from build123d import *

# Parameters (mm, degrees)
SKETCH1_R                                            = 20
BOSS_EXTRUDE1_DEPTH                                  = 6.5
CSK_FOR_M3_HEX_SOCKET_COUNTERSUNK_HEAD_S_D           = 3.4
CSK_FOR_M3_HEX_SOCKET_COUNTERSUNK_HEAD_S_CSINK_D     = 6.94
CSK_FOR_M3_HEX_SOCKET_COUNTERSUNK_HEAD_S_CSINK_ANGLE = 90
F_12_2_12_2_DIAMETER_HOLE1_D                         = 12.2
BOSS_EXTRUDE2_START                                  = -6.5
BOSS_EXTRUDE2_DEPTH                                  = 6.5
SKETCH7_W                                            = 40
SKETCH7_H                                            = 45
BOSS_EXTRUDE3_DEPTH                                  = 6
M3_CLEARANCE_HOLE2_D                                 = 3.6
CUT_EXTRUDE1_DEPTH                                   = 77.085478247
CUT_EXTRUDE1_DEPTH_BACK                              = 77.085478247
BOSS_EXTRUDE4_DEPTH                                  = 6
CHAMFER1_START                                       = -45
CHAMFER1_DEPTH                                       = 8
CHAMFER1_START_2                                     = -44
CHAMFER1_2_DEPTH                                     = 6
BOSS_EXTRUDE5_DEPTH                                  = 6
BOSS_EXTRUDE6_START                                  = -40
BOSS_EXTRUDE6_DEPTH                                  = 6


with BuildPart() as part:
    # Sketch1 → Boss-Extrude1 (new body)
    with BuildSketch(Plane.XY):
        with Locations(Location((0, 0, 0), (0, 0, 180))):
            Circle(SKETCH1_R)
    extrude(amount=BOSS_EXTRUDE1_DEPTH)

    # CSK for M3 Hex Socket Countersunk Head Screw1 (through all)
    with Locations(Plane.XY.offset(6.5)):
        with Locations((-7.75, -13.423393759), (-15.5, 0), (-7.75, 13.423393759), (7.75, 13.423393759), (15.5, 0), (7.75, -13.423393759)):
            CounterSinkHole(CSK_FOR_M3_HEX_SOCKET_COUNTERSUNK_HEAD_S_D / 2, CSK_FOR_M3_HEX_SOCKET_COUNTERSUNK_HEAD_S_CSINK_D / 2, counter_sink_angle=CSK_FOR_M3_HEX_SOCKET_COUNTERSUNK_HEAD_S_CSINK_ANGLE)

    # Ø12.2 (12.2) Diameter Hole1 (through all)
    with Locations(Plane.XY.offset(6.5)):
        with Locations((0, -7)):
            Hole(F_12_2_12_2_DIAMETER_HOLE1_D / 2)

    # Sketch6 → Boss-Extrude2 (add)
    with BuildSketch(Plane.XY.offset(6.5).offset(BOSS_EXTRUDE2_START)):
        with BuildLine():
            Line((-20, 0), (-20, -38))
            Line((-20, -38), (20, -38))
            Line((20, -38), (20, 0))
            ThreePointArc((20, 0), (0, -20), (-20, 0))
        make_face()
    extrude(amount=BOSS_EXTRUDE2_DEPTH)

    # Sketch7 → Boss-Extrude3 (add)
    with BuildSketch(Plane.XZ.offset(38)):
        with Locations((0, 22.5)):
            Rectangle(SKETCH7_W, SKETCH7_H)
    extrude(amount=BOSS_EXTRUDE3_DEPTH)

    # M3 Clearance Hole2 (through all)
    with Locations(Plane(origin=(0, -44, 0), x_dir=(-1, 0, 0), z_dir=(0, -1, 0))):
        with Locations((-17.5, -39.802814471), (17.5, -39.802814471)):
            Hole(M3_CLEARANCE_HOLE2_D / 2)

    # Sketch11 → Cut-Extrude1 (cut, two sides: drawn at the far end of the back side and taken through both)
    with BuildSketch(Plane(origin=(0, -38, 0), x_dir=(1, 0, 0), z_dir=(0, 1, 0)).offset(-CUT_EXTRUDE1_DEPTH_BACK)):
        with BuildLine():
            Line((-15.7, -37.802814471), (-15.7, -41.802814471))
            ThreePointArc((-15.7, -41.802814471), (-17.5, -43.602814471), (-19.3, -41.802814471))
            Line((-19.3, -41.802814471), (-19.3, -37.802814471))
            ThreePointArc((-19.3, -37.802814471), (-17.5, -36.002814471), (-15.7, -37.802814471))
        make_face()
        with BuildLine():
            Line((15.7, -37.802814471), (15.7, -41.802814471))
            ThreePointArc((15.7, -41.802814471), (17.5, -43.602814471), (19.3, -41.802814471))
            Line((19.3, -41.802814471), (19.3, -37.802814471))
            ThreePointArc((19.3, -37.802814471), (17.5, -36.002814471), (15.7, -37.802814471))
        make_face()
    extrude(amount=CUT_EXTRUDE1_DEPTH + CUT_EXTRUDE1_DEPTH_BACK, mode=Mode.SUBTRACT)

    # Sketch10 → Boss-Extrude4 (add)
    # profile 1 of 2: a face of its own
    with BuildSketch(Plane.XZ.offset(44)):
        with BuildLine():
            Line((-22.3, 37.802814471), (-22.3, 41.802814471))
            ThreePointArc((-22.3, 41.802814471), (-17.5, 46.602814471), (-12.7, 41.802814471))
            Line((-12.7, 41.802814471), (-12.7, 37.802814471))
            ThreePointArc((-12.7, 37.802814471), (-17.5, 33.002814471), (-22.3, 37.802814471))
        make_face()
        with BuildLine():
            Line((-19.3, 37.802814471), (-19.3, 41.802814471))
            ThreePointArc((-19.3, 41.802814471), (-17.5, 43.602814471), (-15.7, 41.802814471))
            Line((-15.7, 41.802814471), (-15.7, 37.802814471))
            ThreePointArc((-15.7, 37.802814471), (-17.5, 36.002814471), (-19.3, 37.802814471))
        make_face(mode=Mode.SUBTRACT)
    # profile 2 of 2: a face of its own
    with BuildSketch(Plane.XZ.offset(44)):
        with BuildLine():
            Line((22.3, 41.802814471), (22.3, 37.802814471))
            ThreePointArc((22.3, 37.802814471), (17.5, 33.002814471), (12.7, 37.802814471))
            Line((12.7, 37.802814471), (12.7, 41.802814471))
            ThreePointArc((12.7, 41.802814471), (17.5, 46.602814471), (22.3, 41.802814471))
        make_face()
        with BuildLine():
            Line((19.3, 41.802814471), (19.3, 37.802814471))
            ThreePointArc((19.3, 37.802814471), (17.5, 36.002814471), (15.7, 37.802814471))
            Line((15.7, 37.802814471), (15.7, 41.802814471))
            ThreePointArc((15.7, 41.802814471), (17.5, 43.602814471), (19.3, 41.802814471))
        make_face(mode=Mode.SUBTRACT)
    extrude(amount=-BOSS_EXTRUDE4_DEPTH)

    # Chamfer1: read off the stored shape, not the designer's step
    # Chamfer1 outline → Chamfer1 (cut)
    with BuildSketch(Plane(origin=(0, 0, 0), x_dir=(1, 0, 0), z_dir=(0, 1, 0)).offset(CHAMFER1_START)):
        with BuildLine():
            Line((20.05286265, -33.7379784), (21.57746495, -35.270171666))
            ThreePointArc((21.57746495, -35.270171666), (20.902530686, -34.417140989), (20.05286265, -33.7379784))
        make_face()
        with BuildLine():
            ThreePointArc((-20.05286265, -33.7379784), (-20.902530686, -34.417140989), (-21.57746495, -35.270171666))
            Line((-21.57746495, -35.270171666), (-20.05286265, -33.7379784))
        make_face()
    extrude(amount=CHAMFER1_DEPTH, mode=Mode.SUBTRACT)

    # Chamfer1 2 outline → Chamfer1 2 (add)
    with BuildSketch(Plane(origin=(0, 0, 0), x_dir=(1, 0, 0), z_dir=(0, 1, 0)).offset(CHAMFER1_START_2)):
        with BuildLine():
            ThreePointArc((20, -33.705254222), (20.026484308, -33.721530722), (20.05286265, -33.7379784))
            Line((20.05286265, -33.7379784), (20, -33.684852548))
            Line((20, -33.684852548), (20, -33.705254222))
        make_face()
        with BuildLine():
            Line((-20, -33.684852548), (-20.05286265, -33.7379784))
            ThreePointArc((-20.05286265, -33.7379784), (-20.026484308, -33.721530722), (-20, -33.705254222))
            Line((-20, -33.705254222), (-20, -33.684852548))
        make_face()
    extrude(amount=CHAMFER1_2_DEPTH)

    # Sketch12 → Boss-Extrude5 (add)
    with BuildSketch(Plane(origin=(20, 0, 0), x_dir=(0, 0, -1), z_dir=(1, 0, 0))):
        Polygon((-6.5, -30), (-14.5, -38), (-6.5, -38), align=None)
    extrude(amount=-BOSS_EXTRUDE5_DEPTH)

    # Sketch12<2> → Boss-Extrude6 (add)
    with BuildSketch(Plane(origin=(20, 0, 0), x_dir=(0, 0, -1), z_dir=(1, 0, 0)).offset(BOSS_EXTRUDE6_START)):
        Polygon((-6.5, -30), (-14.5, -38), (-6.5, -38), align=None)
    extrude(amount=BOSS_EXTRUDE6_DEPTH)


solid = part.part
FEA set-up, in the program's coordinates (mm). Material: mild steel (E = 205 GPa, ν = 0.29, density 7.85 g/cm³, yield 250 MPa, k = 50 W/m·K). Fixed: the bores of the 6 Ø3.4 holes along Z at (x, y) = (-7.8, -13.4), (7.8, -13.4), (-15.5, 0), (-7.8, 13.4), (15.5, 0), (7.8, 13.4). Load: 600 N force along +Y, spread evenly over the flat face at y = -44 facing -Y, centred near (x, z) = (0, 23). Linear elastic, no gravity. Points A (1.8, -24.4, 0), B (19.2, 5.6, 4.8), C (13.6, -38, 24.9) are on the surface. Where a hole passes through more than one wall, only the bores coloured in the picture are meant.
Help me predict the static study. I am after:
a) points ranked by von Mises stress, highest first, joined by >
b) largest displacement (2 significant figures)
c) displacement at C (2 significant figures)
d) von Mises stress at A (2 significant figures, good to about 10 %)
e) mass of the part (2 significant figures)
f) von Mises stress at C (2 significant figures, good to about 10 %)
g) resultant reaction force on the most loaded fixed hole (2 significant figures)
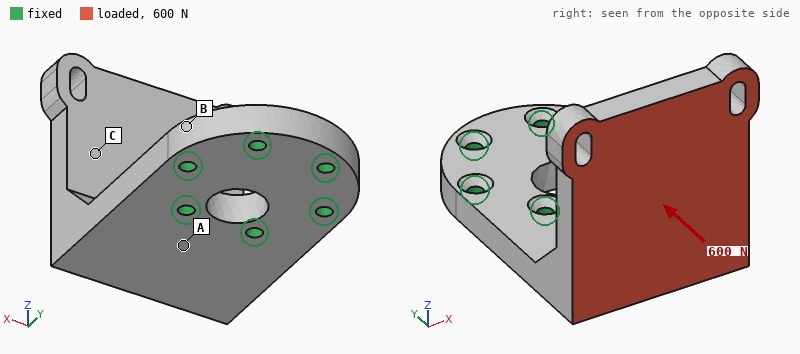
A > C > B
99 µm
47 µm
32 MPa
190 g
13 MPa
260 N
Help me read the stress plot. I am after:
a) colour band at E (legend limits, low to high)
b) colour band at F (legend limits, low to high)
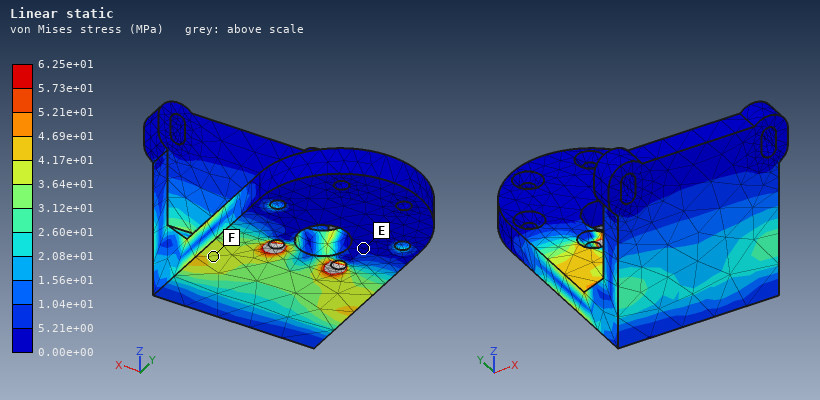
0.00e+00 to 5.21e+00 MPa
3.64e+01 to 4.17e+01 MPa
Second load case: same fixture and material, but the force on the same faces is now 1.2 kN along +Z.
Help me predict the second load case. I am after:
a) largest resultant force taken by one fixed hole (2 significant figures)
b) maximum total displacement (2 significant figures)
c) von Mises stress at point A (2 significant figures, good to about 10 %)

1.2 kN
0.17 mm
70 MPa
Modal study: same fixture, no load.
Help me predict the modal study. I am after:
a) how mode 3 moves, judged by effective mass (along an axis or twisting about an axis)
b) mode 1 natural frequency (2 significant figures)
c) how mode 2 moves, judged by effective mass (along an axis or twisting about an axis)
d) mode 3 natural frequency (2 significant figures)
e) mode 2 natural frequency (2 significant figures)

along Z
1500 Hz
along X
4300 Hz
2500 Hz
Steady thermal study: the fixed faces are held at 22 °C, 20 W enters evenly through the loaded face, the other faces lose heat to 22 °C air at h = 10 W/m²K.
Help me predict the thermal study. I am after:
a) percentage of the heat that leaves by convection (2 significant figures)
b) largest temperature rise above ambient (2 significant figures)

10 %
64 K
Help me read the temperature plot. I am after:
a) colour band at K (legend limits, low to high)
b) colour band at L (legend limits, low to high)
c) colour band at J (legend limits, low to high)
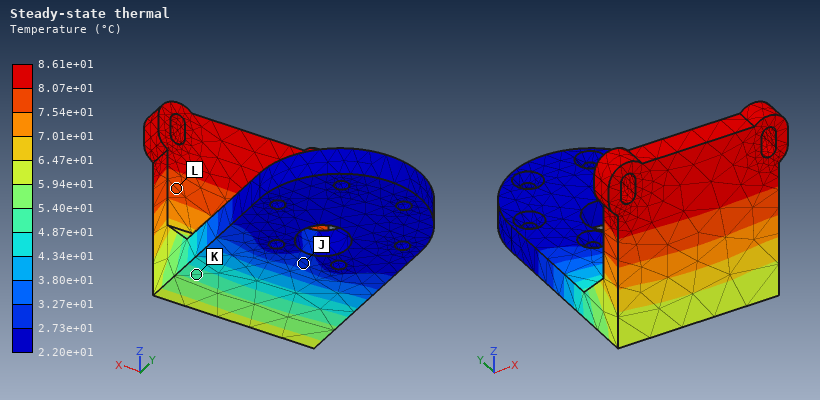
4.87e+01 to 5.40e+01 °C
7.54e+01 to 8.07e+01 °C
2.73e+01 to 3.27e+01 °C
